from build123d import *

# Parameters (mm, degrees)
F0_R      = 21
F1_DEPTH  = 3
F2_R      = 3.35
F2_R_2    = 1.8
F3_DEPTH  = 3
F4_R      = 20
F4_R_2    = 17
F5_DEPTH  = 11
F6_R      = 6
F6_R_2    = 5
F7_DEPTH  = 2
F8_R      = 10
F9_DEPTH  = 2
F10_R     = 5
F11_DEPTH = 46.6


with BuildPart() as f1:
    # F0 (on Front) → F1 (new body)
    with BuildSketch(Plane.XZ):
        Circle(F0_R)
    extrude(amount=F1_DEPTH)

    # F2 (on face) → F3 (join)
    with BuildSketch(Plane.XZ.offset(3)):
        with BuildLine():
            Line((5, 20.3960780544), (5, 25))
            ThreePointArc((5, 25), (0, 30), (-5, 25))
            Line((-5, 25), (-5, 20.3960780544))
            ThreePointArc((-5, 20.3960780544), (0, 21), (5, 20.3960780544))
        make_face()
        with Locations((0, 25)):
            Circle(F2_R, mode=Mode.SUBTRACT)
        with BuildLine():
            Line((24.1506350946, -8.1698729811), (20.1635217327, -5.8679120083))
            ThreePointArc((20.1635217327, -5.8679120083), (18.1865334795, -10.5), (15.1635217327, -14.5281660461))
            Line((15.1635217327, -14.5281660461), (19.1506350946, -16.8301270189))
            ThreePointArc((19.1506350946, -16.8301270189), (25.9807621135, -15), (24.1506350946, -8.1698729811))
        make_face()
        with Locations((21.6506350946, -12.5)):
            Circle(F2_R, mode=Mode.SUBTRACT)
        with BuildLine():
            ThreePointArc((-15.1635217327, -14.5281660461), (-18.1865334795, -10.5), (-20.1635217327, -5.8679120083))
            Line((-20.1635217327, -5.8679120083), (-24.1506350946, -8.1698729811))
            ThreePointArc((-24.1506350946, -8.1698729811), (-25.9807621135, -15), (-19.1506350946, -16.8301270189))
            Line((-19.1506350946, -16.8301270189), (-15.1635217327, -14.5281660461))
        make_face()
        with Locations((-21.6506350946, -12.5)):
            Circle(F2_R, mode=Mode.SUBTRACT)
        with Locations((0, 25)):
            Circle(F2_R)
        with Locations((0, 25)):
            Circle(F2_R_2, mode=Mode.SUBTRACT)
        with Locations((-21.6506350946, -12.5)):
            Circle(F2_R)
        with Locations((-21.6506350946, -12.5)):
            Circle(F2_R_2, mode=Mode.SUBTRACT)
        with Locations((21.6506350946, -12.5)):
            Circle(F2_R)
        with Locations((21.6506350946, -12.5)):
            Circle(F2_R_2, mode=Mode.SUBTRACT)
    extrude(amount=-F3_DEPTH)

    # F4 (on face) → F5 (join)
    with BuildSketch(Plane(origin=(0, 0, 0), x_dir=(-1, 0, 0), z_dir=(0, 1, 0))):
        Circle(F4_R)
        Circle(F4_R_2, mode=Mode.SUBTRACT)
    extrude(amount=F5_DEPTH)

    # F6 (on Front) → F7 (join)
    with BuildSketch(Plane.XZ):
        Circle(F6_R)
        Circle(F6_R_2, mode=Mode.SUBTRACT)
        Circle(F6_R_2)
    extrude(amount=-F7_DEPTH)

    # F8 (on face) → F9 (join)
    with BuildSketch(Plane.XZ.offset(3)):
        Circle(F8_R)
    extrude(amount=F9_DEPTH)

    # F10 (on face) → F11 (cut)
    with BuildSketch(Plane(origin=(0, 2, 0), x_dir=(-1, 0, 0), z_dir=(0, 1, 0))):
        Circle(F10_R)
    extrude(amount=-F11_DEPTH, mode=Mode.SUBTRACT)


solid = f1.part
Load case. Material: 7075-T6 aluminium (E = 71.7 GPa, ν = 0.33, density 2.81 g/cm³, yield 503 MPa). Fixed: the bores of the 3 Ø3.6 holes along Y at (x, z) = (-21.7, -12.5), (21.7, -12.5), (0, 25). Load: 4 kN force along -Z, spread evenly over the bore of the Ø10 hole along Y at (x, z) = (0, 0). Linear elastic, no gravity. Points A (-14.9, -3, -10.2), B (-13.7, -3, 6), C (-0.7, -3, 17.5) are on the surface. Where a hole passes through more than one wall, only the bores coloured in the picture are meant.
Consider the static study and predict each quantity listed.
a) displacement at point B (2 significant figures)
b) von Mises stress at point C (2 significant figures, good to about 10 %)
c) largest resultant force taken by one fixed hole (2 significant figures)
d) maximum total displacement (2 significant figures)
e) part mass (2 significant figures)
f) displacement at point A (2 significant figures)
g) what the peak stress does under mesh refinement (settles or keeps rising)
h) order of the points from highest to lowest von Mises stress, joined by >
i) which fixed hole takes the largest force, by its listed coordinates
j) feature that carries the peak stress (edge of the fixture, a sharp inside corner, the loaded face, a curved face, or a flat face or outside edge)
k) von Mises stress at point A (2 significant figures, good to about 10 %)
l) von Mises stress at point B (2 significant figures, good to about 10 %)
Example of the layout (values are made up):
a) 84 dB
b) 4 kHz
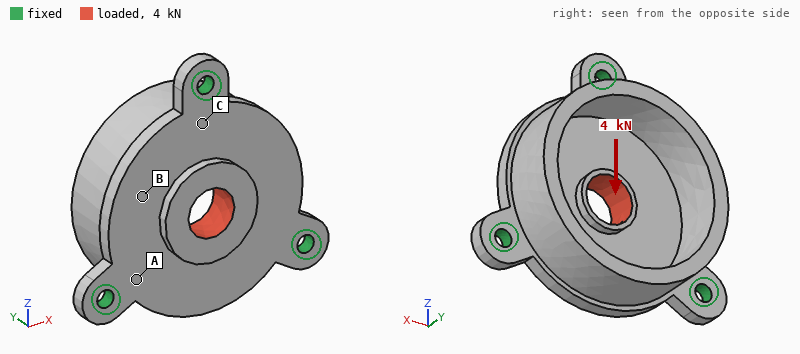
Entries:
a) 11 µm
b) 59 MPa
c) 1.8 kN
d) 30 µm
e) 25 g
f) 8.7 µm
g) keeps rising
h) C > A > B
i) (0, 25)
j) edge of the fixture
k) 31 MPa
l) 13 MPa
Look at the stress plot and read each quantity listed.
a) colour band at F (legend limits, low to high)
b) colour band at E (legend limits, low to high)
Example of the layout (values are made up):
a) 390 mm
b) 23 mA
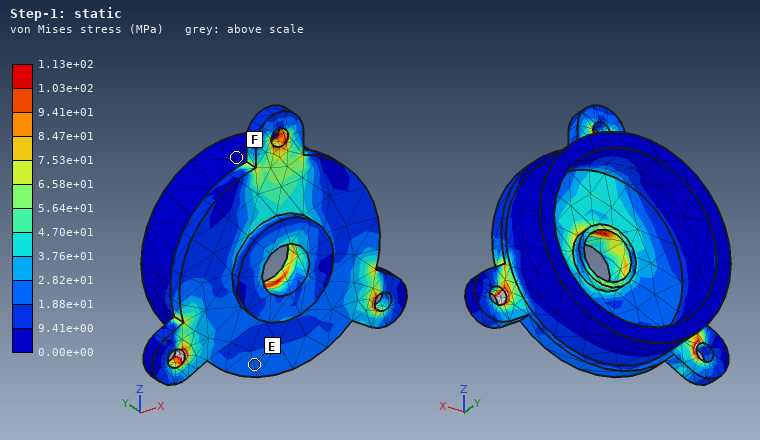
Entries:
a) 0.00e+00 to 9.41e+00 MPa
b) 1.88e+01 to 2.82e+01 MPa
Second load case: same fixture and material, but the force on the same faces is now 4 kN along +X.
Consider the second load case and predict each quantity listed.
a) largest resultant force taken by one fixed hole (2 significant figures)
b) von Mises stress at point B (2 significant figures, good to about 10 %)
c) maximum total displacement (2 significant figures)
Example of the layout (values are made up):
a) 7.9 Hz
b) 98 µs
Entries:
a) 1.6 kN
b) 16 MPa
c) 27 µm
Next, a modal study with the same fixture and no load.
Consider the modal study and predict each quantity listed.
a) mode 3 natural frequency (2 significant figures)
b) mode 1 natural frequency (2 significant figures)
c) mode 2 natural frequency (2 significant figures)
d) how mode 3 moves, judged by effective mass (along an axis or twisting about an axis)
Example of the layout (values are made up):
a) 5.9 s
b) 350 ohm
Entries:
a) 9800 Hz
b) 8100 Hz
c) 8100 Hz
d) along Y
